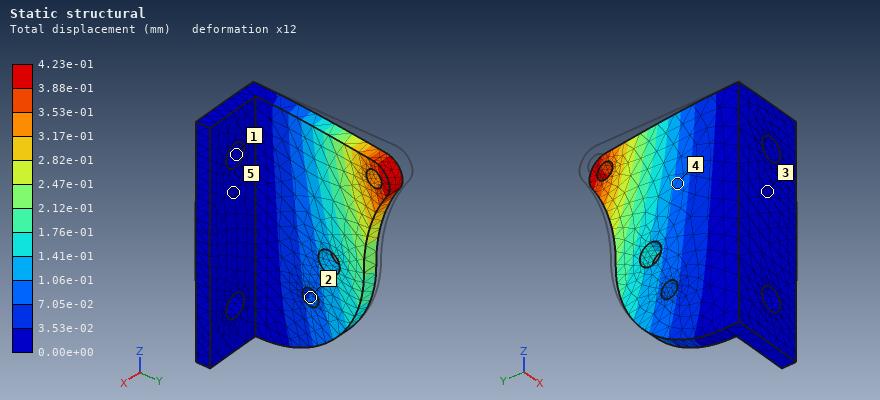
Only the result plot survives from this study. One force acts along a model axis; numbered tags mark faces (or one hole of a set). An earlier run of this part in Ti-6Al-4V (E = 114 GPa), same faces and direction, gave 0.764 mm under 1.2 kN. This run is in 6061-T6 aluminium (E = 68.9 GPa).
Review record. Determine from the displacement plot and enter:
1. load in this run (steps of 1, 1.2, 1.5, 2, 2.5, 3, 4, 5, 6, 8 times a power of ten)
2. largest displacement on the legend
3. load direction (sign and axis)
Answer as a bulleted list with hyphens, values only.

- 400 N
- 4.23e-01 mm
- +X
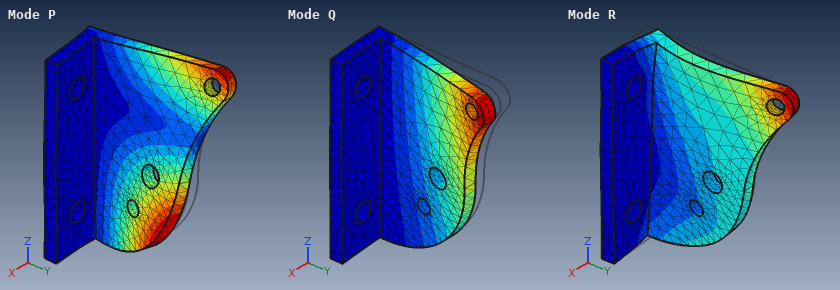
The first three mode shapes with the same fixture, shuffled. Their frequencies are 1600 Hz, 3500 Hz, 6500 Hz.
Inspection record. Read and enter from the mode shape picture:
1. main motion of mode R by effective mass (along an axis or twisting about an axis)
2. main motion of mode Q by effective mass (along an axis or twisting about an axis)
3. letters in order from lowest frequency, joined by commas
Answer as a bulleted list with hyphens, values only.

- along Z
- along X
- Q, P, R
